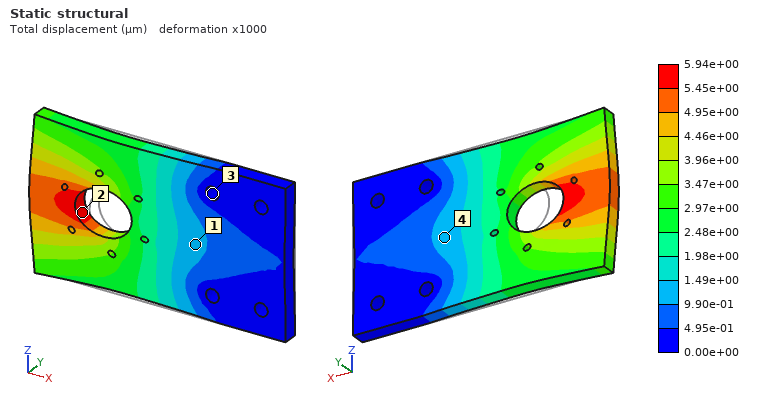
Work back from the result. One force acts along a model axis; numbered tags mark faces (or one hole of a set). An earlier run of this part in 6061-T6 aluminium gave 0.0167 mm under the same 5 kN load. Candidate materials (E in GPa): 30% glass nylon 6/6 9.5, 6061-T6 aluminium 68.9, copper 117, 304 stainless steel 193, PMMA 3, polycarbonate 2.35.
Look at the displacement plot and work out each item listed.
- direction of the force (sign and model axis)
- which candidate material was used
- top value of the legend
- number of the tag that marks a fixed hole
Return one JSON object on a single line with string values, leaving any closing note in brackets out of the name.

{"direction of the force": "-X", "which candidate material was used": "304 stainless steel", "top value of the legend": "5.94e+00 µm", "number of the tag that marks a fixed hole": "3"}
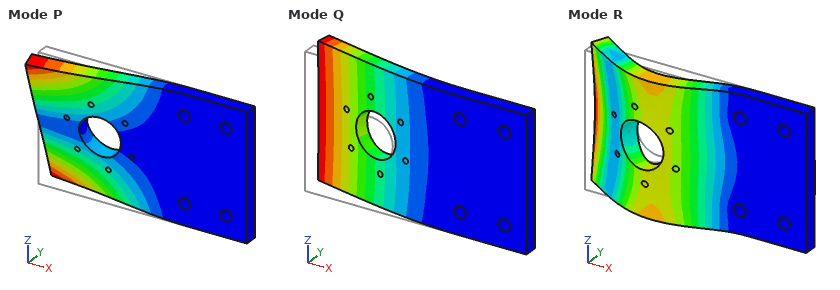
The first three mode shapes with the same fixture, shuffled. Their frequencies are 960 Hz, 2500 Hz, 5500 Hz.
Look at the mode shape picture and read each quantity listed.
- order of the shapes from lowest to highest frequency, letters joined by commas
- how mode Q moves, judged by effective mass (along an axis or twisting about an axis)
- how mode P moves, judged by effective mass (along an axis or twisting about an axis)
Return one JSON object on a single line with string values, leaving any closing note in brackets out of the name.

{"order of the shapes from lowest to highest frequency, letters joined by commas": "Q, P, R", "how mode Q moves, judged by effective mass": "along Y", "how mode P moves, judged by effective mass": "twisting about X"}
